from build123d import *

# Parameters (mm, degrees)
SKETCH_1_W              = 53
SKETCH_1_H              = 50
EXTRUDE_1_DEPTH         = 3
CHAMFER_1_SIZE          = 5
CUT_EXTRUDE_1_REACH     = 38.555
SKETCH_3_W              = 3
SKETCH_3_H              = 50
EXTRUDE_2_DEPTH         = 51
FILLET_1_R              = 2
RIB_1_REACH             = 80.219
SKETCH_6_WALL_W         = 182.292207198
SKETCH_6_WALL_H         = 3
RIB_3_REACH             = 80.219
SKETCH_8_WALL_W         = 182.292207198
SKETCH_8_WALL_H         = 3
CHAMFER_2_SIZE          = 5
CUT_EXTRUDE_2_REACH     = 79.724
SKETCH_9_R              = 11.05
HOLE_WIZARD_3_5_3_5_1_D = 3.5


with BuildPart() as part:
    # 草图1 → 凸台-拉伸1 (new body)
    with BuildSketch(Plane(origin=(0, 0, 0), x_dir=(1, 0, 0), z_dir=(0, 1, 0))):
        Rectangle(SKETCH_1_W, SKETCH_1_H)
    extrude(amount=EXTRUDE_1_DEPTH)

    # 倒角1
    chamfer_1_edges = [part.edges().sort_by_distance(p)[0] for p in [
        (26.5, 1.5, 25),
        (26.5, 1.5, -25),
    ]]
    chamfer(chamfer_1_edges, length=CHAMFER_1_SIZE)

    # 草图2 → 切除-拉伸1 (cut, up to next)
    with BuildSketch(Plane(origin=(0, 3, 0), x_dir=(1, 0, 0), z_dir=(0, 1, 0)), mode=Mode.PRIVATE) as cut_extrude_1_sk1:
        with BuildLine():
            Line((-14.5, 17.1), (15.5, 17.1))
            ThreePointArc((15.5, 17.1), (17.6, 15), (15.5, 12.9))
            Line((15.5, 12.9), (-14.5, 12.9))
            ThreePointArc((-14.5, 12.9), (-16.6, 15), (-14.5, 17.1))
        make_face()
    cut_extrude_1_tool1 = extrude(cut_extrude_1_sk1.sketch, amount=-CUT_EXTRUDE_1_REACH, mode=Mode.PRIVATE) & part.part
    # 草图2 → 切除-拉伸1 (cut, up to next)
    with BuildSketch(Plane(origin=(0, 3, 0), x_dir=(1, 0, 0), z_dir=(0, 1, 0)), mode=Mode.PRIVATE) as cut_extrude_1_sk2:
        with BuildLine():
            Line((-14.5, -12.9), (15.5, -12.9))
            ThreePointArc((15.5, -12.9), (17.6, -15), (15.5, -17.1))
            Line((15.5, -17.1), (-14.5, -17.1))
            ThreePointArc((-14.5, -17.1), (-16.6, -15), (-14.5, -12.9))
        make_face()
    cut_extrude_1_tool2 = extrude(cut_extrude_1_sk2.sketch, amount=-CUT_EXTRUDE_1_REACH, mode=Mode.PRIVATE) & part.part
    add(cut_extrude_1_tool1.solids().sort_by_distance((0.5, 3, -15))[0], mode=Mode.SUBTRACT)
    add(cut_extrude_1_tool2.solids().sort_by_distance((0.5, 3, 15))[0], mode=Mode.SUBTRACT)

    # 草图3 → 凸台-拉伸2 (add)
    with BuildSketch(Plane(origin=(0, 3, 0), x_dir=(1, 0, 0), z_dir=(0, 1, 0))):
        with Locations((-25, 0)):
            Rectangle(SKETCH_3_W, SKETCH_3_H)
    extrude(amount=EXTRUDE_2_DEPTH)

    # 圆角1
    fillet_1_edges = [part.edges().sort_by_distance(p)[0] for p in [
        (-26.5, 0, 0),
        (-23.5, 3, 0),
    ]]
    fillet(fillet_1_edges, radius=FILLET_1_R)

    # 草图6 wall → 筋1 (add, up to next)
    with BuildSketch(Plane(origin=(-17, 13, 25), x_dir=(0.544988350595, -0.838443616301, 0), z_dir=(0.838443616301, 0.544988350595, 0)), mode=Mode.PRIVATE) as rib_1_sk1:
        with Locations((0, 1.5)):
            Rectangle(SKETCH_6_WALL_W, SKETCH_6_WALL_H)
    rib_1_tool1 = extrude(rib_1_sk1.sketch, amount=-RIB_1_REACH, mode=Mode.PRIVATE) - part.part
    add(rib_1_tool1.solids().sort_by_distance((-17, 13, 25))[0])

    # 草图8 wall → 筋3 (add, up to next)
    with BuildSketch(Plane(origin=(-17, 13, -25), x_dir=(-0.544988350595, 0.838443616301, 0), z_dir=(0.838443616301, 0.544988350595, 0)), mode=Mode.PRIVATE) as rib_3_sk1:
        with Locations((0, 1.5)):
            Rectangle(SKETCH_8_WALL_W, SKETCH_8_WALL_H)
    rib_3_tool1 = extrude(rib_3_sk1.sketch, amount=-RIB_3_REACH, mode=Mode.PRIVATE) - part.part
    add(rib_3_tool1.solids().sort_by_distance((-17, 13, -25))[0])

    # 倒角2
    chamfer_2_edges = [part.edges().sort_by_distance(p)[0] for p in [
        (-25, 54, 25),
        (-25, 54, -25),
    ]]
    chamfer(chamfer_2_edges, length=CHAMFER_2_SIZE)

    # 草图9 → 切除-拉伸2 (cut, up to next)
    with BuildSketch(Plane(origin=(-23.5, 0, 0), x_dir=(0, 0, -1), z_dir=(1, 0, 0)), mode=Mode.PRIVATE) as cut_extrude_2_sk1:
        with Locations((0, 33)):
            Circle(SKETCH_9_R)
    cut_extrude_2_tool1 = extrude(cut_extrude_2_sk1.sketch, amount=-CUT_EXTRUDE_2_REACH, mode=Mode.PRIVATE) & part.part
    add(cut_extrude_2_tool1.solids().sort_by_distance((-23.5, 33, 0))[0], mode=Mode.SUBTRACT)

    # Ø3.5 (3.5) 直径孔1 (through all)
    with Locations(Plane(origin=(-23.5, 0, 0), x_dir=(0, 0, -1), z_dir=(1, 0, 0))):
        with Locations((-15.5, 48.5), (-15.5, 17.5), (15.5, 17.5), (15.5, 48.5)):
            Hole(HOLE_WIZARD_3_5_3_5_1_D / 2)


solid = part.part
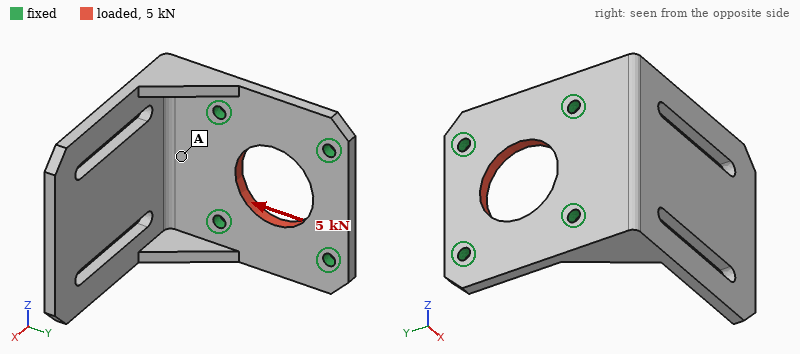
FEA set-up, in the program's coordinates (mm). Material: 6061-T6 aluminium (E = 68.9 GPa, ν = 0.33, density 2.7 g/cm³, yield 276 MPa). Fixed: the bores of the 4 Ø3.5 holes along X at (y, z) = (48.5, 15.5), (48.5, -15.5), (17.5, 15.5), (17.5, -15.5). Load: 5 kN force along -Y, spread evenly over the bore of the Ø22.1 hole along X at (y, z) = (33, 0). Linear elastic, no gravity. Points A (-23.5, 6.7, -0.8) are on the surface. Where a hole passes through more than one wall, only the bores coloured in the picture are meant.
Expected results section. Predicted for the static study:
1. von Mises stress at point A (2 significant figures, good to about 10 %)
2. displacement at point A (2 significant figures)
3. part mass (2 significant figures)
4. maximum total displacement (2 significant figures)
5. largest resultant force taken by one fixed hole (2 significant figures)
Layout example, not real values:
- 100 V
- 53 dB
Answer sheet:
- 8.8 MPa
- 5.2 µm
- 38 g
- 15 µm
- 1.3 kN
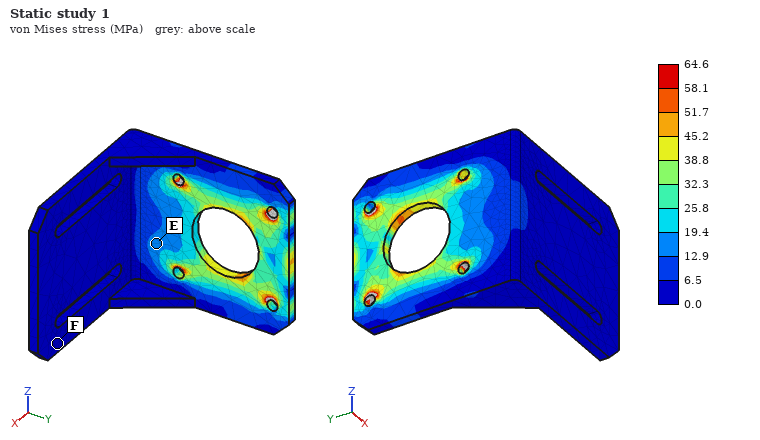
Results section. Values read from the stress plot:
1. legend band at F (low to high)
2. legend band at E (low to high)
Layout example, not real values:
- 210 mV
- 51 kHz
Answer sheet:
- 0.0 to 6.5 MPa
- 12.9 to 19.4 MPa
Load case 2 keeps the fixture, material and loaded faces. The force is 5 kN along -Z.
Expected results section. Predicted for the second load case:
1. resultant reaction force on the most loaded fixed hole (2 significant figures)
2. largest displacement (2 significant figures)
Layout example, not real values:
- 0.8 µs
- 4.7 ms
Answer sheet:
- 1.3 kN
- 12 µm
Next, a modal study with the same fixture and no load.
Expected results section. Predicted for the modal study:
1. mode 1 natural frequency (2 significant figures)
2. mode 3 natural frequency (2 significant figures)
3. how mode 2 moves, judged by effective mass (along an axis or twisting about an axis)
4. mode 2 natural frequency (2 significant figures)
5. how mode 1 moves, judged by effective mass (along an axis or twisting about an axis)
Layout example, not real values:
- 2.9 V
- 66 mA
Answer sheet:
- 910 Hz
- 3100 Hz
- along Z
- 1900 Hz
- along Y
